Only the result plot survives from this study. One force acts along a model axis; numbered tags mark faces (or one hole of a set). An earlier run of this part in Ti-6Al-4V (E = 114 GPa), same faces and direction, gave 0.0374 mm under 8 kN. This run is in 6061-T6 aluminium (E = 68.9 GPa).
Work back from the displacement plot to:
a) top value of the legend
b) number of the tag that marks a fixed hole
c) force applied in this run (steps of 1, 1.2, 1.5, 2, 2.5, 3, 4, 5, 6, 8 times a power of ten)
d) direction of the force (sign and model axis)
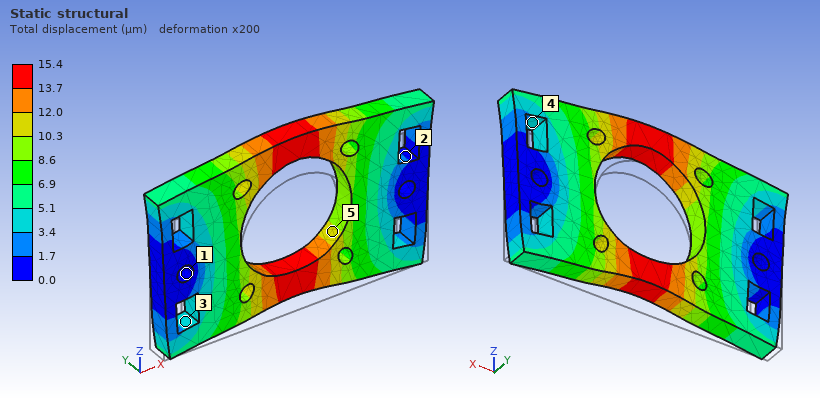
15.4 µm
1
2 kN
+Z
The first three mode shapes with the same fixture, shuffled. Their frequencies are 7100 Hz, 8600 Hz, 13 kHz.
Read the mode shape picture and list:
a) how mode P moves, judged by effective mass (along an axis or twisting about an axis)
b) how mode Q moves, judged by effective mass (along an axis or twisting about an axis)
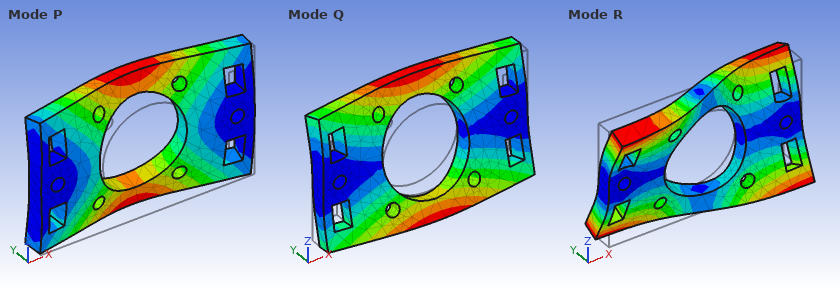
along Y
twisting about X
